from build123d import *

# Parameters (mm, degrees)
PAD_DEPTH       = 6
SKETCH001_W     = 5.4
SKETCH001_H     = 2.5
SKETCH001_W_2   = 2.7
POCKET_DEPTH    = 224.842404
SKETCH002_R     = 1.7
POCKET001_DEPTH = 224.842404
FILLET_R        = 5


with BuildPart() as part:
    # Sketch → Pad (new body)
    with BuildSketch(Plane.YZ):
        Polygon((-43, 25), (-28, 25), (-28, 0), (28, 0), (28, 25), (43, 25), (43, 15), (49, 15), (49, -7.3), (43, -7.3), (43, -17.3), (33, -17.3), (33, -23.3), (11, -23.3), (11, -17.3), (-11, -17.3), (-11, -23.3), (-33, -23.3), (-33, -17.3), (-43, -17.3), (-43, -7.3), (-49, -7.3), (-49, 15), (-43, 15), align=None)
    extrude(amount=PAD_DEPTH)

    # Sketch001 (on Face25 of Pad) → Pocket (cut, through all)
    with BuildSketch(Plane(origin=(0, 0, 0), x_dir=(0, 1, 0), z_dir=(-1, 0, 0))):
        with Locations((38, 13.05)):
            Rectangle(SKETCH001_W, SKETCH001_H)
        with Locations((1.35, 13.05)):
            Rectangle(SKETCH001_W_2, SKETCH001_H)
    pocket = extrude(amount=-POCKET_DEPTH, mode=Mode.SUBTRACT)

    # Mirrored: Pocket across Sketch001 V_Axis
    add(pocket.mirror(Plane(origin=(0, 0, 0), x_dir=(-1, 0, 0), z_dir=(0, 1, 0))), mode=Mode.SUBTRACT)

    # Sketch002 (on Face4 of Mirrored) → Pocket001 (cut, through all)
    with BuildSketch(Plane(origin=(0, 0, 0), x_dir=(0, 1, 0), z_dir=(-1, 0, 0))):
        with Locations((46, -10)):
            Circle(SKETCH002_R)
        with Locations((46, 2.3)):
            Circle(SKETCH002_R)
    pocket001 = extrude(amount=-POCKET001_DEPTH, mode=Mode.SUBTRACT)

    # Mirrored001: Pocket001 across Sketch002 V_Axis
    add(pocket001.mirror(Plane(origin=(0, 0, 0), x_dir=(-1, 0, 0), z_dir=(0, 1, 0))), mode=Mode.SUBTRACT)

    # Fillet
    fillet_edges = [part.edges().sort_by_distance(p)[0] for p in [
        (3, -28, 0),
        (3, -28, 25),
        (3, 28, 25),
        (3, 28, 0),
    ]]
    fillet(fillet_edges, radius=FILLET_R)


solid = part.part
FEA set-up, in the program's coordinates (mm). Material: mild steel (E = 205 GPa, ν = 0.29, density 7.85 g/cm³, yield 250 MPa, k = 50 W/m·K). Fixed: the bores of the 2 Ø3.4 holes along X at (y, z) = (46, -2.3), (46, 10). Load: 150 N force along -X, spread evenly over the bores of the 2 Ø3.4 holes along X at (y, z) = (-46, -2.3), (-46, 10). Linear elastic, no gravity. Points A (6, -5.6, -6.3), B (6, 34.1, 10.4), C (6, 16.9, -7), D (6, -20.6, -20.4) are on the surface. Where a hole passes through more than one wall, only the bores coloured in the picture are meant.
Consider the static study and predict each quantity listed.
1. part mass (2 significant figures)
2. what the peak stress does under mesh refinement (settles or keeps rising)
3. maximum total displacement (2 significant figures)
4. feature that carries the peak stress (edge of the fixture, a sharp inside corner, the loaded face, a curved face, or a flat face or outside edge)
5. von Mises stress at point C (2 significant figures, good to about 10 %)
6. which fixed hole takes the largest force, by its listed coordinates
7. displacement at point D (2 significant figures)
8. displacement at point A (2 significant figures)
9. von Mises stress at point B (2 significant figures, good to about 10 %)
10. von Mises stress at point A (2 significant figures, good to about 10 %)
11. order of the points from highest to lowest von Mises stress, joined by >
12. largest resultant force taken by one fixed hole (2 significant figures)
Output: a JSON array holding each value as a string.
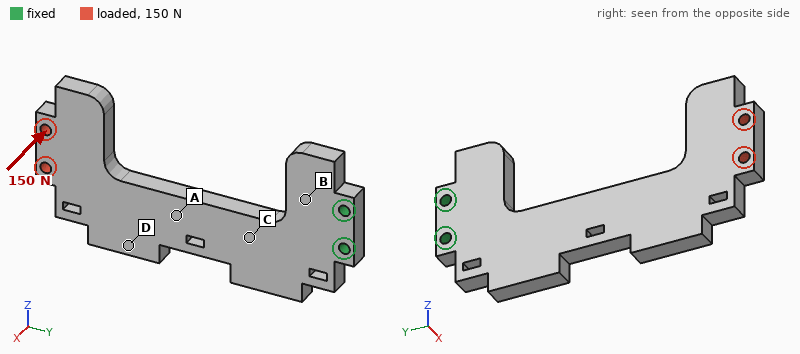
["130 g", "keeps rising", "0.60 mm", "edge of the fixture", "82 MPa", "(46, 10)", "0.31 mm", "0.21 mm", "44 MPa", "64 MPa", "C > A > B > D", "80 N"]
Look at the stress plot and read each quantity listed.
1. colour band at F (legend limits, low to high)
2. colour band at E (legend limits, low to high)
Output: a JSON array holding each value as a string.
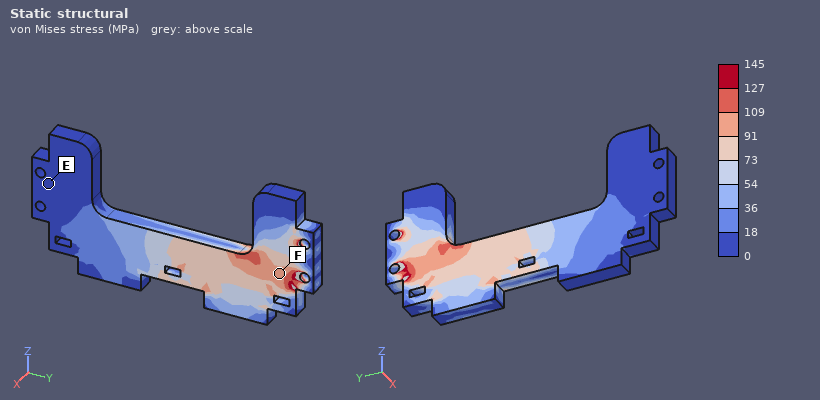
["91 to 109 MPa", "0 to 18 MPa"]
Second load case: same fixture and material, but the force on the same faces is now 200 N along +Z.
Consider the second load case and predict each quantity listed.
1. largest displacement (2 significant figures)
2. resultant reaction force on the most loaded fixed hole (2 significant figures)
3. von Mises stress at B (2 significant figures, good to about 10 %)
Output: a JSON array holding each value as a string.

["92 µm", "1.3 kN", "15 MPa"]
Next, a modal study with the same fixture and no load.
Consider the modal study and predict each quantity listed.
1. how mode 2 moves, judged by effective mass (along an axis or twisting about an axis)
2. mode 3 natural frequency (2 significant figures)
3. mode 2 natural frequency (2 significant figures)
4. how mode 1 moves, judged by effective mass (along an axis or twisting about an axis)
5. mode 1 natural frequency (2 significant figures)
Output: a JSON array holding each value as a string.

["along Z", "1700 Hz", "1300 Hz", "along X", "440 Hz"]
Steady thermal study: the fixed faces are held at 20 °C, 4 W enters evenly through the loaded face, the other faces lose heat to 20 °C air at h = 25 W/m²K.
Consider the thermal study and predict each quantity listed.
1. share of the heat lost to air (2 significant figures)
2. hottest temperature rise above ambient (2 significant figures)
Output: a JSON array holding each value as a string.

["67 %", "34 K"]
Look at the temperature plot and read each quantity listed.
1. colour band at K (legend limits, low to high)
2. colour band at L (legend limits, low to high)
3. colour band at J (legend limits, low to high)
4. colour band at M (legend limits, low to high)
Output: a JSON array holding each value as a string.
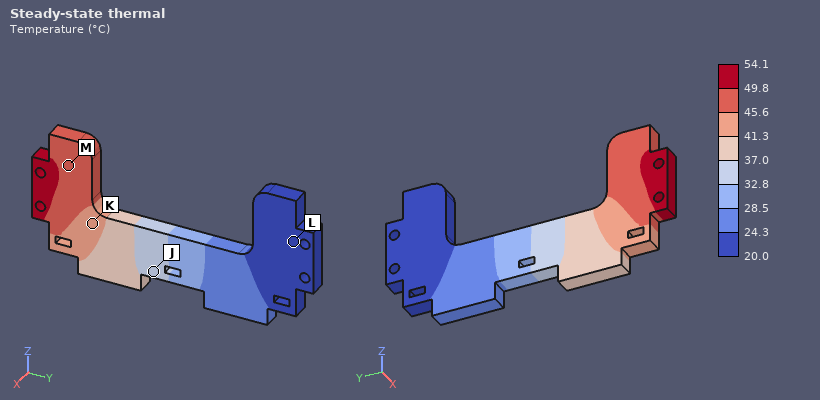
["41.3 to 45.6 °C", "20.0 to 24.3 °C", "32.8 to 37.0 °C", "45.6 to 49.8 °C"]
